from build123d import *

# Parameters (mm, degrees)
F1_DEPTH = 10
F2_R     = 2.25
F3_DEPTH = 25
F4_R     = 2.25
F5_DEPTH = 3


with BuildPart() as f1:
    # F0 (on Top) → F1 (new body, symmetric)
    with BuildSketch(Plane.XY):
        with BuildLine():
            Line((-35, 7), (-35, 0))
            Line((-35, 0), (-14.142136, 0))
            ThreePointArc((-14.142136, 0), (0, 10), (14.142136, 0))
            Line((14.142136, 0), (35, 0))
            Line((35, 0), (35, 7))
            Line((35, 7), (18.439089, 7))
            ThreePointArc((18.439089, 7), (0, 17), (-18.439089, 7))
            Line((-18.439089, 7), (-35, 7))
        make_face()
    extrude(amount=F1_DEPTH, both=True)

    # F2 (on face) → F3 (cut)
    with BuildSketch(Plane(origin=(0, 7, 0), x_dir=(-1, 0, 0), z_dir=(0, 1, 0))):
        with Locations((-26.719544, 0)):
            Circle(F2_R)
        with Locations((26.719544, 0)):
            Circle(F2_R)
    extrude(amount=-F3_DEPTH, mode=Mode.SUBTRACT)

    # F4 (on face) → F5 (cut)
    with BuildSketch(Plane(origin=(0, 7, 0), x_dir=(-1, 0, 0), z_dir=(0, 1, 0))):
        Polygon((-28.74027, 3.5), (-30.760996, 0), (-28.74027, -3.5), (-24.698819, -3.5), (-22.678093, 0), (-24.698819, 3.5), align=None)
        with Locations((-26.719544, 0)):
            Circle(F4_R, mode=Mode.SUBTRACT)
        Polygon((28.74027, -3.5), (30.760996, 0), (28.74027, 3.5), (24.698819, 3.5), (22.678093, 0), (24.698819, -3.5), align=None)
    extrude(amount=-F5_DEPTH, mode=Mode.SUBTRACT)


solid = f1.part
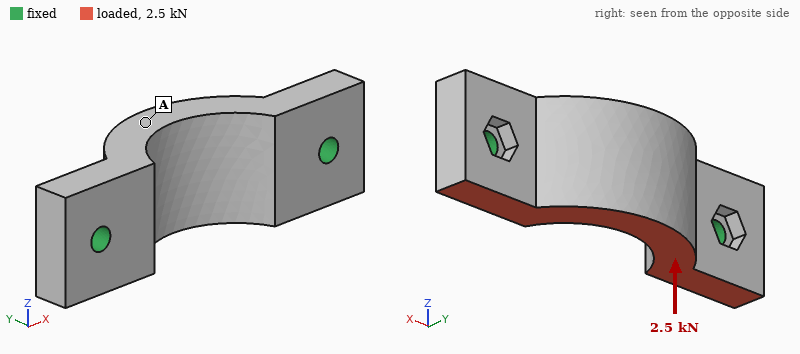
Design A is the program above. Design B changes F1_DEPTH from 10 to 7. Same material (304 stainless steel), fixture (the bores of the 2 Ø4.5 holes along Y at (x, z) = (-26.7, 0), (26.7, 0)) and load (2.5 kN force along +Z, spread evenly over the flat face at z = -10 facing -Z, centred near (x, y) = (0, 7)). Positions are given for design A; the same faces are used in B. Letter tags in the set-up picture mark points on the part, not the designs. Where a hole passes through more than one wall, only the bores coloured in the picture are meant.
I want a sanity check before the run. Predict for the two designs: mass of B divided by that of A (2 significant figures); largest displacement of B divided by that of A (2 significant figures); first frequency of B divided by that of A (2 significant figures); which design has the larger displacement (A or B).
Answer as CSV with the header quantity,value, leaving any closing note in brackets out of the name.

quantity,value
mass of B divided by that of A,0.69
largest displacement of B divided by that of A,1.2
first frequency of B divided by that of A,1.1
which design has the larger displacement,B
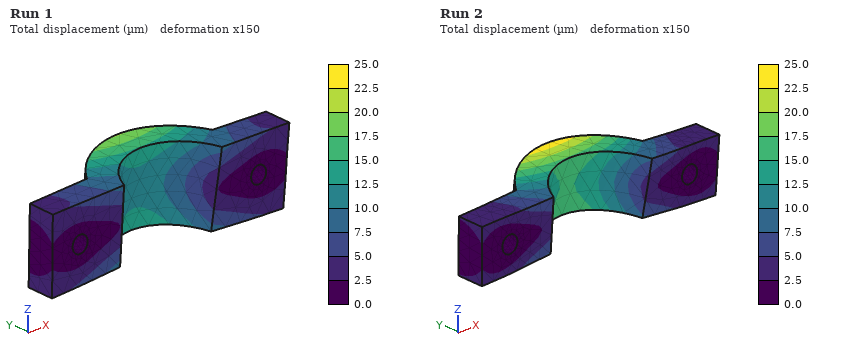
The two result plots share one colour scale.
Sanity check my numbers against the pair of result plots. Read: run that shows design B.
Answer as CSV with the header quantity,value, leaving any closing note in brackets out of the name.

quantity,value
run that shows design B,Run 2
